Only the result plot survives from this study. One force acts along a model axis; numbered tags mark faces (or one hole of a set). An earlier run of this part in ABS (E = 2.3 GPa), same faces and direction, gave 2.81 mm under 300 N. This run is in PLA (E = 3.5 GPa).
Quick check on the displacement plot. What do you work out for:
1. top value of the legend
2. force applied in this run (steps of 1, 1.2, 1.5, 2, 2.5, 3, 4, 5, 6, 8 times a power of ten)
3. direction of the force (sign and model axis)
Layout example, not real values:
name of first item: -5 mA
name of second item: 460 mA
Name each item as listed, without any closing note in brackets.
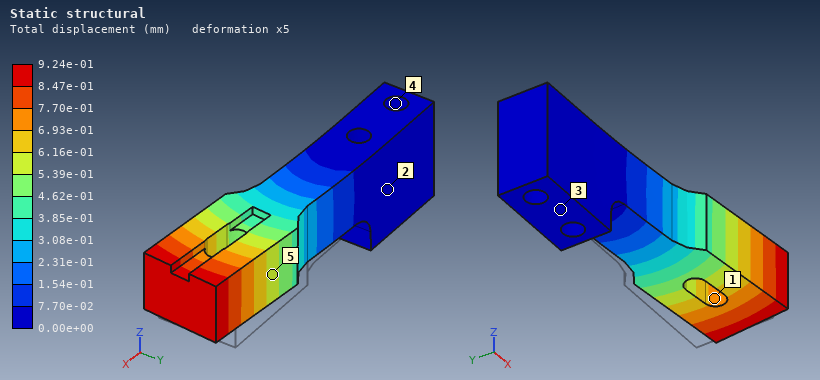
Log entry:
top value of the legend: 9.24e-01 mm
force applied in this run: 150 N
direction of the force: -Y
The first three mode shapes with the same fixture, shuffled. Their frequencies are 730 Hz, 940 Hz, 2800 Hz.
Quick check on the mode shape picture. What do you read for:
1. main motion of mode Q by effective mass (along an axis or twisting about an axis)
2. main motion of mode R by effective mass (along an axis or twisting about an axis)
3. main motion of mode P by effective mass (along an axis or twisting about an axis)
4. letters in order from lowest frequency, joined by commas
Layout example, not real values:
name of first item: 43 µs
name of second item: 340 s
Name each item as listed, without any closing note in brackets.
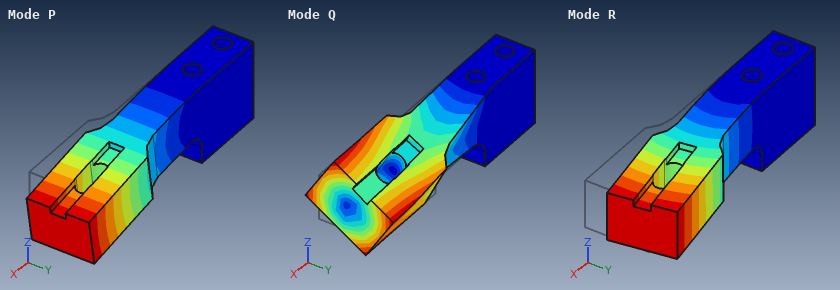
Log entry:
main motion of mode Q by effective mass: twisting about X
main motion of mode R by effective mass: along Y
main motion of mode P by effective mass: along Z
letters in order from lowest frequency, joined by commas: R, P, Q
